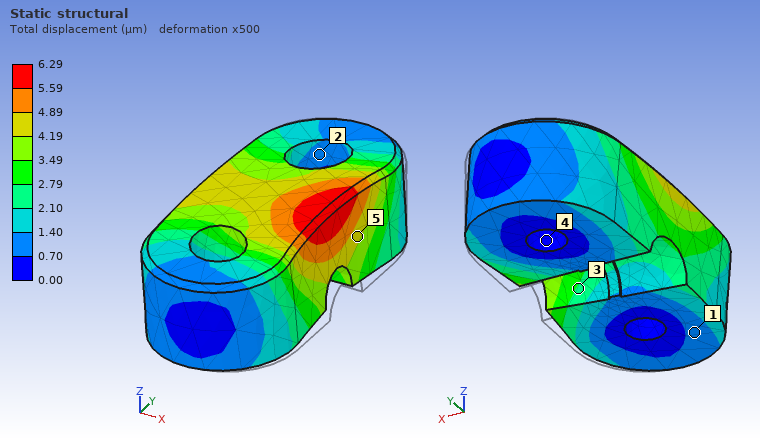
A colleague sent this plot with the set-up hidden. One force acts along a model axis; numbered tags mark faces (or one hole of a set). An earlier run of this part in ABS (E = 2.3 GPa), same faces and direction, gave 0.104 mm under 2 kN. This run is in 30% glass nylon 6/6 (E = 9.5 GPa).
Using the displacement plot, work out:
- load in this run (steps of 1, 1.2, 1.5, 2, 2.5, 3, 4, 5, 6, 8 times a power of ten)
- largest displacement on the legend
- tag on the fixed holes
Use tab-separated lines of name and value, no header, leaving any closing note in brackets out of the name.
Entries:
load in this run	500 N
largest displacement on the legend	6.29 µm
tag on the fixed holes	4
